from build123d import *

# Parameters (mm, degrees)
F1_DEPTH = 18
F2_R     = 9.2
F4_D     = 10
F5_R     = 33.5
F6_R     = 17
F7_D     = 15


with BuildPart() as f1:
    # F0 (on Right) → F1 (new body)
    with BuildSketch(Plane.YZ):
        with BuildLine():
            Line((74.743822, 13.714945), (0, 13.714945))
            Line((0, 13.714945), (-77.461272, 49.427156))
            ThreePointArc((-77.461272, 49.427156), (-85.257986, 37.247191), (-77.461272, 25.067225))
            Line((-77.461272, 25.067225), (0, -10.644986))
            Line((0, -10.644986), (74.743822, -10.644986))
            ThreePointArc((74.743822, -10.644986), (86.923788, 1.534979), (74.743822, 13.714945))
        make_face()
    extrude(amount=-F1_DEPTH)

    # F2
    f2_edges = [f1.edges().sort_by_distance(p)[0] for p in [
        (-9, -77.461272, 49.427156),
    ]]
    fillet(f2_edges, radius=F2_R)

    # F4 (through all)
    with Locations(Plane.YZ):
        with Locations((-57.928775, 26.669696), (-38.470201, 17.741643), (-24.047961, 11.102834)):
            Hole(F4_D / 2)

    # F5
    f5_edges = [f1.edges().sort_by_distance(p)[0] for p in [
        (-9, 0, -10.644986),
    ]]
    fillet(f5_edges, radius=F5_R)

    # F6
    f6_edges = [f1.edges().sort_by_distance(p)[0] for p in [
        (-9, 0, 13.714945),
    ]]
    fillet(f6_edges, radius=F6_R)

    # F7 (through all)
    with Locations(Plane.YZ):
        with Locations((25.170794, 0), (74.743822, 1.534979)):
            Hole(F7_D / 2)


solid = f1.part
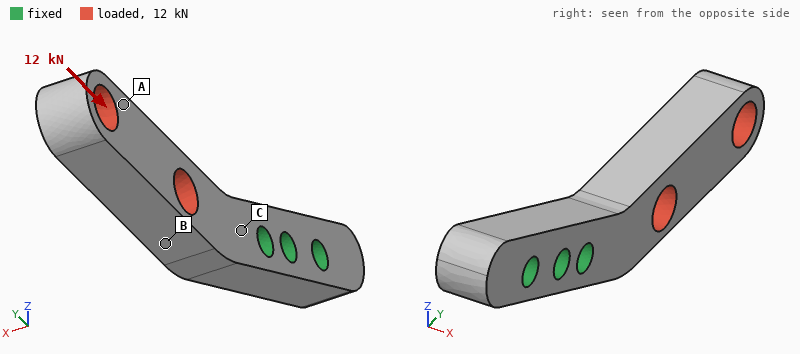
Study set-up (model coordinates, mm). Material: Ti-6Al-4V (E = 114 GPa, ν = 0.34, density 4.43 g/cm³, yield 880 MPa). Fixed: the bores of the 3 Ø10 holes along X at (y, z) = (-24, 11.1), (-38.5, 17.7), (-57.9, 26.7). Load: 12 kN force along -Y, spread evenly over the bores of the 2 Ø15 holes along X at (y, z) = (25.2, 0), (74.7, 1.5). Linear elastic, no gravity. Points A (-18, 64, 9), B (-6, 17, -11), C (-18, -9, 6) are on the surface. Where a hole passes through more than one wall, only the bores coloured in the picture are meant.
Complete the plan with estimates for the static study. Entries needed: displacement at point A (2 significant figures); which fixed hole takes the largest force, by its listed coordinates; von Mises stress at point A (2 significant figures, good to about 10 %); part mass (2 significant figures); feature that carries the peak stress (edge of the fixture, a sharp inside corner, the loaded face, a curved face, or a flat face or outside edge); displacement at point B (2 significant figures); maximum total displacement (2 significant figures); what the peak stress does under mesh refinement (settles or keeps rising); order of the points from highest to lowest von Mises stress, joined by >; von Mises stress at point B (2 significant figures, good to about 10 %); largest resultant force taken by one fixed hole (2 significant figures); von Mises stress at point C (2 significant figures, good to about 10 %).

0.12 mm
(-24, 11.1)
17 MPa
280 g
edge of the fixture
0.062 mm
0.16 mm
keeps rising
B > C > A
72 MPa
13 kN
45 MPa
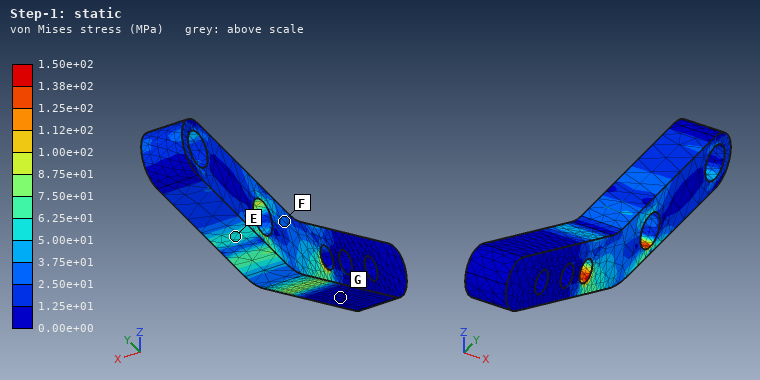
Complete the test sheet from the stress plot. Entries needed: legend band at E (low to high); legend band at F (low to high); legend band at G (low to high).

5.00e+01 to 6.25e+01 MPa
2.50e+01 to 3.75e+01 MPa
0.00e+00 to 1.25e+01 MPa
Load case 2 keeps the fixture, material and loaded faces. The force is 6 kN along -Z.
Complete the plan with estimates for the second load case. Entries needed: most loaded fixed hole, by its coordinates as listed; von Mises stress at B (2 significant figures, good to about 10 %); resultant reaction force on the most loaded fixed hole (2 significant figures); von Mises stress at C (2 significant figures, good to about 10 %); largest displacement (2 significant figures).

(-24, 11.1)
210 MPa
12 kN
45 MPa
0.90 mm
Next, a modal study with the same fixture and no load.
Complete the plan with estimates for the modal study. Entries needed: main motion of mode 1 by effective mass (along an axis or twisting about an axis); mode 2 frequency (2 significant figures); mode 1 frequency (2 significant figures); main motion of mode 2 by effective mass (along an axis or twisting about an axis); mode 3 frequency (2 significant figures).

along X
1500 Hz
1300 Hz
along Z
5800 Hz
